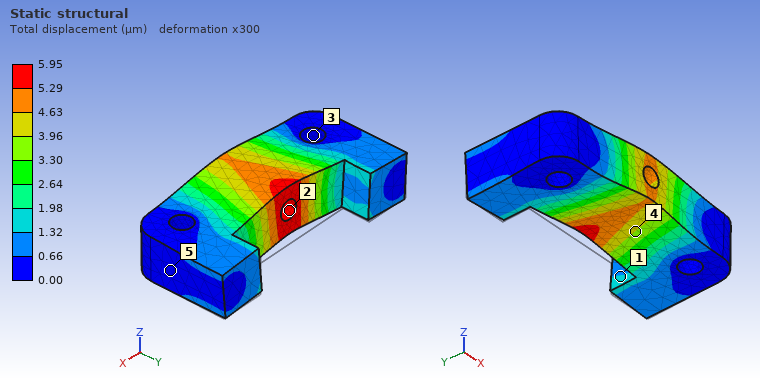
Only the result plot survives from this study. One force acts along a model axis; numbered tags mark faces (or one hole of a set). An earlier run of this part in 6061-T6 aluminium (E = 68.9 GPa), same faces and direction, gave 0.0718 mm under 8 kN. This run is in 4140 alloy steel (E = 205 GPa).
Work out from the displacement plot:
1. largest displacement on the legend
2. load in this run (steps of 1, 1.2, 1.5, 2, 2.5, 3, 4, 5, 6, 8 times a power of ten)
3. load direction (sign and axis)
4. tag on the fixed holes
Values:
5.95 µm
2 kN
+Z
3
